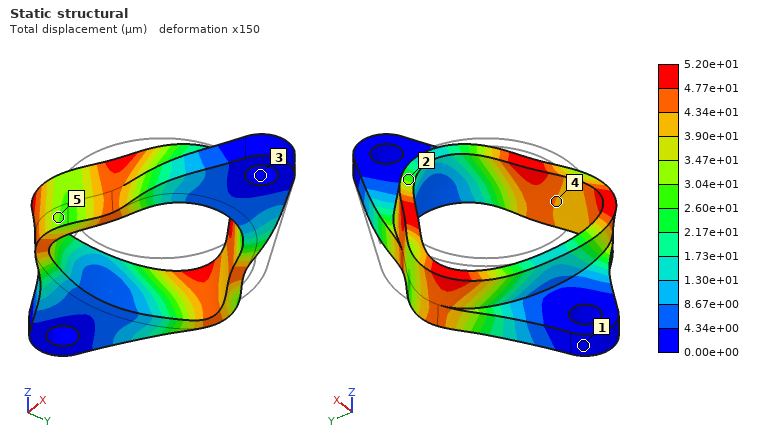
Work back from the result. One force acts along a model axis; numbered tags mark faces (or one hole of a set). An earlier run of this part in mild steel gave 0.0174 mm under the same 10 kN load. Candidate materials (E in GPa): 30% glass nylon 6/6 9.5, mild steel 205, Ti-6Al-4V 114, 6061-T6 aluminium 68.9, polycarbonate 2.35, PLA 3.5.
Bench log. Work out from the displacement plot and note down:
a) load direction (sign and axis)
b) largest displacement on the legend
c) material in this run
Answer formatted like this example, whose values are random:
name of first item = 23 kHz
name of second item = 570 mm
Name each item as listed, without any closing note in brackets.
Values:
load direction = -X
largest displacement on the legend = 5.20e+01 µm
material in this run = 6061-T6 aluminium
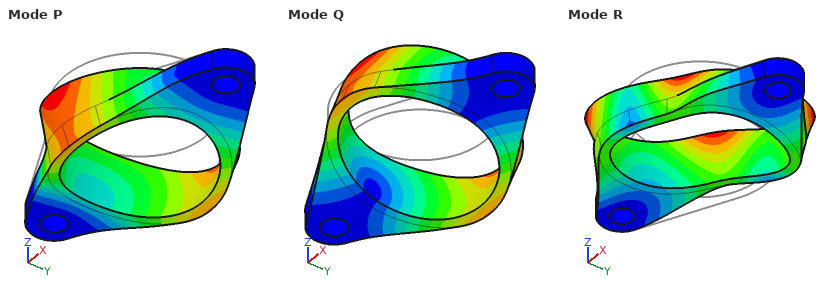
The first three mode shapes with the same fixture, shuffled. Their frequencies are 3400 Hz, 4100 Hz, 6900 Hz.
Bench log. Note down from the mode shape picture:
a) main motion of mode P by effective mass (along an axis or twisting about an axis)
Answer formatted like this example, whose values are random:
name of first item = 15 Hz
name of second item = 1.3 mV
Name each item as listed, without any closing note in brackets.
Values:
main motion of mode P by effective mass = along Z
